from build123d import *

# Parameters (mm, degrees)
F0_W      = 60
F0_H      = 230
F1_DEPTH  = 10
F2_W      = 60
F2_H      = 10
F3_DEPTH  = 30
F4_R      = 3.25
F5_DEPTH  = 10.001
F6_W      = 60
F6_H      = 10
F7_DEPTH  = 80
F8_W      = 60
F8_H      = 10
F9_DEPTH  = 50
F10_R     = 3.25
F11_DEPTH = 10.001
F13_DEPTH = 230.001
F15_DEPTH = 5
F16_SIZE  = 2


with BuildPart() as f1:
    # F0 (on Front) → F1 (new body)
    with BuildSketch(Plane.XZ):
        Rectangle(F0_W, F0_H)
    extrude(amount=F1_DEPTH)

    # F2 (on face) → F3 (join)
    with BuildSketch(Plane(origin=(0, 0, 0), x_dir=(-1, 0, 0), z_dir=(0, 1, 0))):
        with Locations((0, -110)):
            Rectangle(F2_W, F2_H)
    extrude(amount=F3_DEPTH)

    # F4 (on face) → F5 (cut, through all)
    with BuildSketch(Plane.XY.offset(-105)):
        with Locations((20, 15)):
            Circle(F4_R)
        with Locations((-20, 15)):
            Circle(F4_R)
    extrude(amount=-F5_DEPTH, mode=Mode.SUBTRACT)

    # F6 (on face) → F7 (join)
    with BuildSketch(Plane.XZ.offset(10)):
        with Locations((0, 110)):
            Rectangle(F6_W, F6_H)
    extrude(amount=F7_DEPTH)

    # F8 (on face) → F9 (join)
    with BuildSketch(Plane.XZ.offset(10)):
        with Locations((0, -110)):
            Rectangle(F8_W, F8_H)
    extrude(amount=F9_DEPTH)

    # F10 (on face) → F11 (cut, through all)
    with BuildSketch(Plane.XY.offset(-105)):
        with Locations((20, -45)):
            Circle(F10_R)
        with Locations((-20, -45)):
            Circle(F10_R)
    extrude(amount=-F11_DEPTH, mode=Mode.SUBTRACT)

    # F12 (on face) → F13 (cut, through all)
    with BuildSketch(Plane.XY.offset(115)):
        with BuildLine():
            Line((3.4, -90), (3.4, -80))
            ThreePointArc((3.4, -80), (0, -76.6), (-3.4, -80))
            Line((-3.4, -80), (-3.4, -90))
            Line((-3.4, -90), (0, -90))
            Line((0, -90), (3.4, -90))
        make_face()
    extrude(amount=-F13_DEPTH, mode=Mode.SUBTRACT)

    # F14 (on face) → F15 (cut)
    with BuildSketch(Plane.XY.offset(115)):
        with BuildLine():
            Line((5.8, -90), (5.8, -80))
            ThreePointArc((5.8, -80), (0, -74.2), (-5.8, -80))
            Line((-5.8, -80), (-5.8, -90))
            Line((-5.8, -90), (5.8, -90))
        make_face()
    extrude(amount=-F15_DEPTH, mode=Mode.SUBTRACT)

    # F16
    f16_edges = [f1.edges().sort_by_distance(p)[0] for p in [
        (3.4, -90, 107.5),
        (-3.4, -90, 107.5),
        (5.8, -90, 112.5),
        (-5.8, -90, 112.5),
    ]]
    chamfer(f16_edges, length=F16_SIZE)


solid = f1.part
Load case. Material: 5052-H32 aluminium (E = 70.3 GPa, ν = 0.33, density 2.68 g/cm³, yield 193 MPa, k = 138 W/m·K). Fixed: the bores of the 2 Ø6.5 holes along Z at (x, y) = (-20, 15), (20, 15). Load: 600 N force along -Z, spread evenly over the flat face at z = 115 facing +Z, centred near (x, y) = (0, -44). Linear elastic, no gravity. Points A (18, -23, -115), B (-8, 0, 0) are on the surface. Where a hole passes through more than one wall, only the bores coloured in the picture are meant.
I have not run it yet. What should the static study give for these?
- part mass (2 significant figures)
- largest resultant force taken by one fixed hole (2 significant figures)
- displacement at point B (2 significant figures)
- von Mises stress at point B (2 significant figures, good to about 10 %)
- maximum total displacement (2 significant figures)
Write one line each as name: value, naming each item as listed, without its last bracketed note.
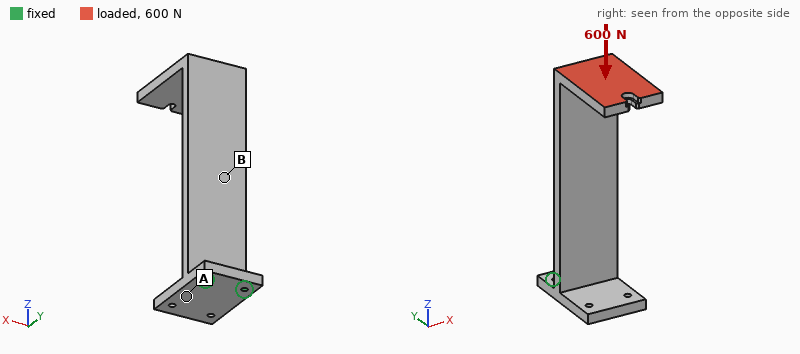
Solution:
part mass: 620 g
largest resultant force taken by one fixed hole: 310 N
displacement at point B: 0.55 mm
von Mises stress at point B: 22 MPa
maximum total displacement: 2.5 mm
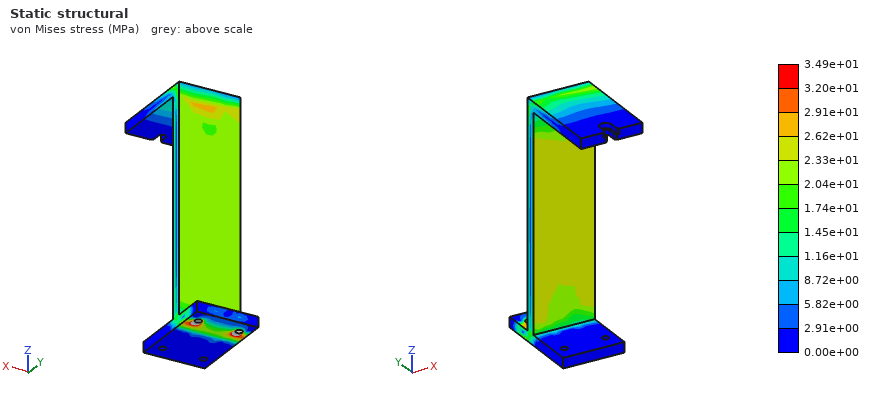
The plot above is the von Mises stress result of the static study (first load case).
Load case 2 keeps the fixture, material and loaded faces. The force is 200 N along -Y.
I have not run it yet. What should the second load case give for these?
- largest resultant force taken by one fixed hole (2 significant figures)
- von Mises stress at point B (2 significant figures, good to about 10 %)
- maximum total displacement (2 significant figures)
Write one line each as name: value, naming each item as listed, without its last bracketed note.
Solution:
largest resultant force taken by one fixed hole: 160 N
von Mises stress at point B: 23 MPa
maximum total displacement: 2.9 mm
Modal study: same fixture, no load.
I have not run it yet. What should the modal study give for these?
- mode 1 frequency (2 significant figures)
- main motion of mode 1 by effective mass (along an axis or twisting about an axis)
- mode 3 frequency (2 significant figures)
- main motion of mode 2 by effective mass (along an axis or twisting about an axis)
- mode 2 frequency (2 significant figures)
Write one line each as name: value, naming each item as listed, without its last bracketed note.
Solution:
mode 1 frequency: 94 Hz
main motion of mode 1 by effective mass: along Y
mode 3 frequency: 520 Hz
main motion of mode 2 by effective mass: along X
mode 2 frequency: 320 Hz
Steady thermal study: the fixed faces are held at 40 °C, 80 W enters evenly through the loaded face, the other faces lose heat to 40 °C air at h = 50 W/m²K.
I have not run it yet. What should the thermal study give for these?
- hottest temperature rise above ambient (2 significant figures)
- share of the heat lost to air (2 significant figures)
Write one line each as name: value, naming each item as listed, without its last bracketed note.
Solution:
hottest temperature rise above ambient: 84 K
share of the heat lost to air: 87 %
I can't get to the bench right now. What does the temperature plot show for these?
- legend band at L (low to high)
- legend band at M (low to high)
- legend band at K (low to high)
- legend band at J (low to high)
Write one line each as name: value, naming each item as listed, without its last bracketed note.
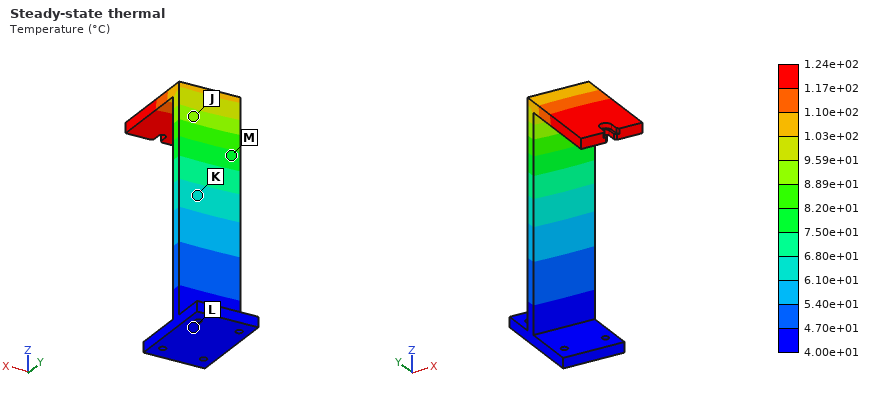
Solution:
legend band at L: 4.00e+01 to 4.70e+01 °C
legend band at M: 7.50e+01 to 8.20e+01 °C
legend band at K: 6.10e+01 to 6.80e+01 °C
legend band at J: 8.89e+01 to 9.59e+01 °C
